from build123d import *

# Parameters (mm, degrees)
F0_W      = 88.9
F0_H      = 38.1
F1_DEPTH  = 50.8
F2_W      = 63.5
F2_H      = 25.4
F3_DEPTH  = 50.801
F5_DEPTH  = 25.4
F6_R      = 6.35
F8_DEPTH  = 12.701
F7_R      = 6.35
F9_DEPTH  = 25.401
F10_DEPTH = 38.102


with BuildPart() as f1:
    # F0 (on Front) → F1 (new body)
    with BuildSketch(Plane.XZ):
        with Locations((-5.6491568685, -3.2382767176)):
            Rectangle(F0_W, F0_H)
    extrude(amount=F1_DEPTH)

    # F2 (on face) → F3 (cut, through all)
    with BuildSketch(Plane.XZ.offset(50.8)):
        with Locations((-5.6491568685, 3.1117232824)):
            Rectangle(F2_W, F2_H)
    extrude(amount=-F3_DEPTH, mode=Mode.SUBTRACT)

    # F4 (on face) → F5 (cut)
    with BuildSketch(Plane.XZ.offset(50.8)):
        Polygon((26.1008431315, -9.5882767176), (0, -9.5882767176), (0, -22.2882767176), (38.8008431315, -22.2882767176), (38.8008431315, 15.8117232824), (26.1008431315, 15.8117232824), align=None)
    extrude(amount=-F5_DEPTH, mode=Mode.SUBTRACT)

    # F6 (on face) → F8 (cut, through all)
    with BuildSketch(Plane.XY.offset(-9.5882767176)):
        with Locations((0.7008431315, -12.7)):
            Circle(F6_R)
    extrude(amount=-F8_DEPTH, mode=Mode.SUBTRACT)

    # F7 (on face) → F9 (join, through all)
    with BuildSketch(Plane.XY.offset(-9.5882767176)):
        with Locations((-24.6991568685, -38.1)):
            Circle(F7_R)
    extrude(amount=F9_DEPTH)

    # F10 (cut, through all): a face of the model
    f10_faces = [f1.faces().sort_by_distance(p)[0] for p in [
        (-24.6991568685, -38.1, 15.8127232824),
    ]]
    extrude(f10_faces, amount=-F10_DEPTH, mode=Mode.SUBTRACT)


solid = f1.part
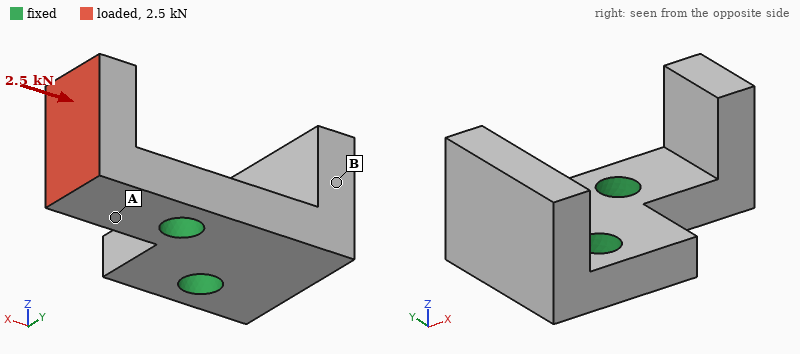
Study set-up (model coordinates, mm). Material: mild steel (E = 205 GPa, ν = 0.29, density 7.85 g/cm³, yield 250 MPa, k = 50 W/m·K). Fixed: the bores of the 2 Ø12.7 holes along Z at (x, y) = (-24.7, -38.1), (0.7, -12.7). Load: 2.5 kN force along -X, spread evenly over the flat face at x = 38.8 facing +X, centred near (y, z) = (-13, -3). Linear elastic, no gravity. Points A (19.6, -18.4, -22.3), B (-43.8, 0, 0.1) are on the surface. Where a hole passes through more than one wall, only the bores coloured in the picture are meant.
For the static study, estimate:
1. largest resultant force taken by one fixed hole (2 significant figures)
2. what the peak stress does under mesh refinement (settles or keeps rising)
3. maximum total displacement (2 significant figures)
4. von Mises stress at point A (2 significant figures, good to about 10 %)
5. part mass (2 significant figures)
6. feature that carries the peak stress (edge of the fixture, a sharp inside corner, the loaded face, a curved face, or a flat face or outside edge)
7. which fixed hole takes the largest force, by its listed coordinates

2.4 kN
keeps rising
43 µm
38 MPa
520 g
edge of the fixture
(0.7, -12.7)
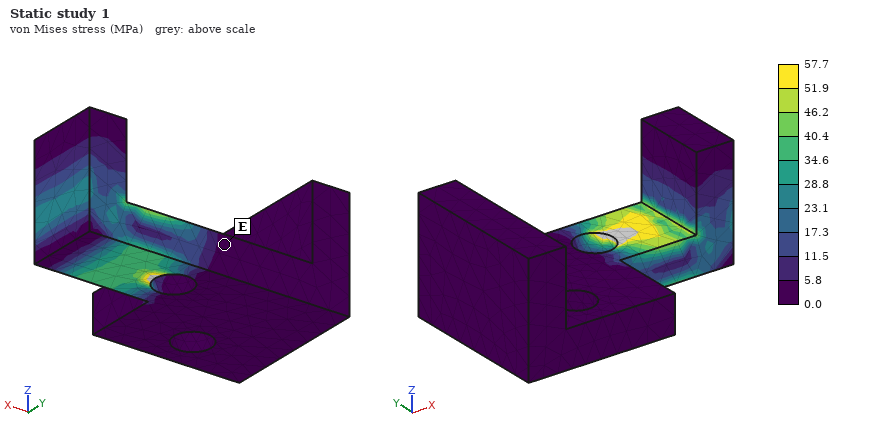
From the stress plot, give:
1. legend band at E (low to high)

0.0 to 5.8 MPa
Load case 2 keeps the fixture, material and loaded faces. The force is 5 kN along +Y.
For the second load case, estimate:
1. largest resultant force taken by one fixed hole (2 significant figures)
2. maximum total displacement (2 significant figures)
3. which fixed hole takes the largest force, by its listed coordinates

5.6 kN
86 µm
(0.7, -12.7)
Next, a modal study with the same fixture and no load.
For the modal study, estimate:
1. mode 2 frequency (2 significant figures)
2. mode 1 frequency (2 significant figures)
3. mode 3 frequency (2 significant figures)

4700 Hz
3800 Hz
4900 Hz
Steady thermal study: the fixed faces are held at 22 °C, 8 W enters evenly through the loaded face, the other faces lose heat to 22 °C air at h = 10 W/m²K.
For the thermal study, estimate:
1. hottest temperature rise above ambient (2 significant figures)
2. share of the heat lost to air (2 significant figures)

18 K
5.3 %
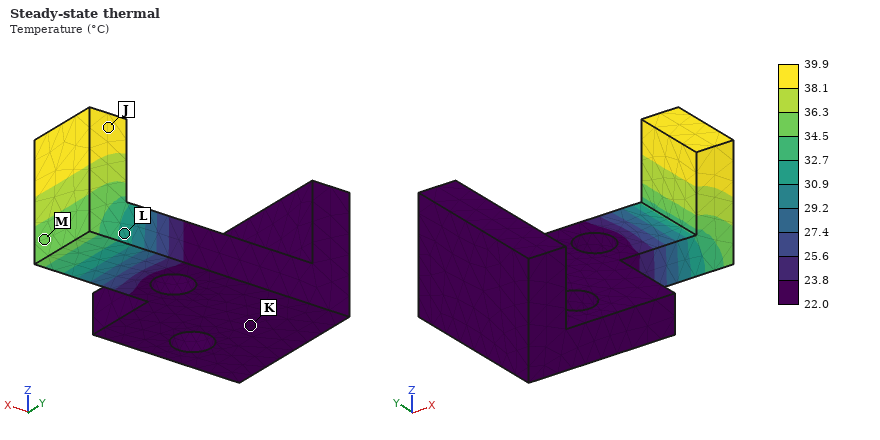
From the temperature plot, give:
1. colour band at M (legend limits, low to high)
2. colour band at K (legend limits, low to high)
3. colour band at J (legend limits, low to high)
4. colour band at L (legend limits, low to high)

34.5 to 36.3 °C
22.0 to 23.8 °C
38.1 to 39.9 °C
30.9 to 32.7 °C
